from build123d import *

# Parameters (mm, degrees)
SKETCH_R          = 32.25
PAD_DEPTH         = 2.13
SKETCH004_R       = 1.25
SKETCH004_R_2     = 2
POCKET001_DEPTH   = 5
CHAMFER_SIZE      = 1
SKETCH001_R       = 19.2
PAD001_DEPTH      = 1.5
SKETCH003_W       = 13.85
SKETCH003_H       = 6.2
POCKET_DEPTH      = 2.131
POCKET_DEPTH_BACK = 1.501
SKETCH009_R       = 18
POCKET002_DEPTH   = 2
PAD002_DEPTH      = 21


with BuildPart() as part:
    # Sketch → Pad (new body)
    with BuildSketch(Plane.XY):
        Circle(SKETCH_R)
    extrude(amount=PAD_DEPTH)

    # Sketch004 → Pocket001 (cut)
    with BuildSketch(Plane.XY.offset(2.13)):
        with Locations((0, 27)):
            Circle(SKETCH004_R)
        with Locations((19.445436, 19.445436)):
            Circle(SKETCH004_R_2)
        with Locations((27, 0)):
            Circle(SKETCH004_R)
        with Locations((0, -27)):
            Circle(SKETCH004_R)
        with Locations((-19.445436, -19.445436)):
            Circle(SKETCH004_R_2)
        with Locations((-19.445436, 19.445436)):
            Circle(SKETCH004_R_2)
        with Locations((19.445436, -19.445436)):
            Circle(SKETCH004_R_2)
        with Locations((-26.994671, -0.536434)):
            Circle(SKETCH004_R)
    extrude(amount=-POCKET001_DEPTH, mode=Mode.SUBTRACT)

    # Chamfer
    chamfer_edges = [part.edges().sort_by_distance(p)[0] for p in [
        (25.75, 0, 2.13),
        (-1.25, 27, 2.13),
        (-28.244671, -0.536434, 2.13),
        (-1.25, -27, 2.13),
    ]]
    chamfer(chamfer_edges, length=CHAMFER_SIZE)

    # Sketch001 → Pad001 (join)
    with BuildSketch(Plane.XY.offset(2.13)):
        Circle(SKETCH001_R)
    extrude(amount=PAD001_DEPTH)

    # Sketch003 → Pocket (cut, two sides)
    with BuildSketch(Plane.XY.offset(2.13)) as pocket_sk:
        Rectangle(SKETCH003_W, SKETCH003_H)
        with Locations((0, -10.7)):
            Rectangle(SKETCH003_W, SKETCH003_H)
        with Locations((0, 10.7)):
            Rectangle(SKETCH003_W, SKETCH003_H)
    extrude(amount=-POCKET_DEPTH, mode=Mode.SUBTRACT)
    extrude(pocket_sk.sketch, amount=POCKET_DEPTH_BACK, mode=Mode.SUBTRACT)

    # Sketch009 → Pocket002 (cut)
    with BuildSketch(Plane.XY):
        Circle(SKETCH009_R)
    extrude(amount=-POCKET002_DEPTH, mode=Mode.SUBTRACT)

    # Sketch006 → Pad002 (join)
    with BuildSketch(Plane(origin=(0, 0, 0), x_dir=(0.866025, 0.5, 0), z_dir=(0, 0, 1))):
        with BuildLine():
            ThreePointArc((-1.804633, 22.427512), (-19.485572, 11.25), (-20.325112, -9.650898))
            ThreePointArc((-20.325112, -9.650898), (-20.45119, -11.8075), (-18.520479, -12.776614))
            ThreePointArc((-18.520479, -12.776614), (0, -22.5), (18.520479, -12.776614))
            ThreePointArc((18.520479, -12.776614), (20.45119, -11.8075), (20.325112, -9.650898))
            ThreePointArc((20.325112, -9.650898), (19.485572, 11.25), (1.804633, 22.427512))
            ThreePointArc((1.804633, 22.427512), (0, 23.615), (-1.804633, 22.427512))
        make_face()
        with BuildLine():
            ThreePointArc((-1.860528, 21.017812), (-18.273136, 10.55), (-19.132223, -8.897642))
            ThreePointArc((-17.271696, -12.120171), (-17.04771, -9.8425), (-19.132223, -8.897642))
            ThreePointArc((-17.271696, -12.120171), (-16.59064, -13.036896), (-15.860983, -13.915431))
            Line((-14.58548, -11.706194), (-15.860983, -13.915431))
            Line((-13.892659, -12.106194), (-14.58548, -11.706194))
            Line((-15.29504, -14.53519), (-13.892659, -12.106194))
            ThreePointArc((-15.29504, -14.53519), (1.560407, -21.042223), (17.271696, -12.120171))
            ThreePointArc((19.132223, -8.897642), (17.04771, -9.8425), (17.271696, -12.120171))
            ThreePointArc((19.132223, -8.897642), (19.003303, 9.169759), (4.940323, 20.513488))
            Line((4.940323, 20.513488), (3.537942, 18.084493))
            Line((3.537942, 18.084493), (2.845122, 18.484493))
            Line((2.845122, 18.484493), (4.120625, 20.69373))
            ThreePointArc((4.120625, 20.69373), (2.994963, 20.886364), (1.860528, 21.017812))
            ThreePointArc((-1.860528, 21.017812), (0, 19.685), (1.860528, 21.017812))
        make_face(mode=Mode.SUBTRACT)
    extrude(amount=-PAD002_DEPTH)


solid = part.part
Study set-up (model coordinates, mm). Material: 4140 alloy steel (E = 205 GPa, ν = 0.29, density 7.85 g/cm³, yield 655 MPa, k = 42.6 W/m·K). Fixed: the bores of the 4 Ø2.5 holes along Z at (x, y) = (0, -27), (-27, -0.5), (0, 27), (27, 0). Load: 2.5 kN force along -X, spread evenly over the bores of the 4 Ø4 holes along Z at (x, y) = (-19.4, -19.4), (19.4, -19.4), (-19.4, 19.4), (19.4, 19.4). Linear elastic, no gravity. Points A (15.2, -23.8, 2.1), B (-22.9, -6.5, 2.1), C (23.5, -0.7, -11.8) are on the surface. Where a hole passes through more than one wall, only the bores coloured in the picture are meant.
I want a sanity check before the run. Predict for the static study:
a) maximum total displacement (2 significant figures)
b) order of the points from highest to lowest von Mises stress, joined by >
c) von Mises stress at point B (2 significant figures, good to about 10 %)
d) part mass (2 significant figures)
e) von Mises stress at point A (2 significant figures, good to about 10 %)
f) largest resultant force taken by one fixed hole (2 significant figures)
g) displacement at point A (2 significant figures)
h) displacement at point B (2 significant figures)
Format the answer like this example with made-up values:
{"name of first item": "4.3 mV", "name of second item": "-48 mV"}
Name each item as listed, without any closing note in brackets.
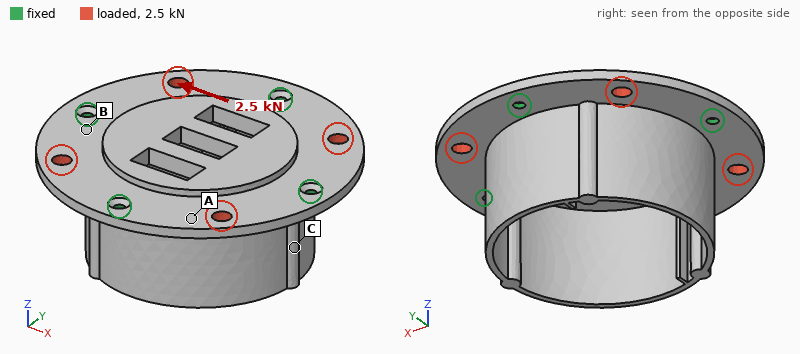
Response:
{"maximum total displacement": "3.0 µm", "order of the points from highest to lowest von Mises stress, joined by >": "A > B > C", "von Mises stress at point B": "11 MPa", "part mass": "95 g", "von Mises stress at point A": "21 MPa", "largest resultant force taken by one fixed hole": "760 N", "displacement at point A": "1.9 µm", "displacement at point B": "1.0 µm"}
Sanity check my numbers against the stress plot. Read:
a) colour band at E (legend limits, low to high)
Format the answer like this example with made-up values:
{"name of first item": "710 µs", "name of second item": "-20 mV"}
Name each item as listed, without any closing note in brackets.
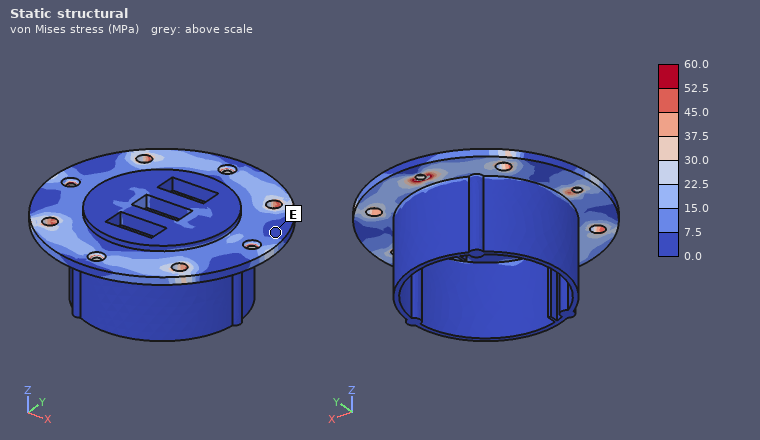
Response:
{"colour band at E": "0.0 to 7.5 MPa"}
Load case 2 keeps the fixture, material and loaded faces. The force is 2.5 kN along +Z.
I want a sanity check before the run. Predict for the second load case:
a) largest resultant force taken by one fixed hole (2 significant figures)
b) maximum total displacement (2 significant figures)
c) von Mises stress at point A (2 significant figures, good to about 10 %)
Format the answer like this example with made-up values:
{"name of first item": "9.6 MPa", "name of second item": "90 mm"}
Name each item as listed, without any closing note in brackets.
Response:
{"largest resultant force taken by one fixed hole": "650 N", "maximum total displacement": "61 µm", "von Mises stress at point A": "82 MPa"}
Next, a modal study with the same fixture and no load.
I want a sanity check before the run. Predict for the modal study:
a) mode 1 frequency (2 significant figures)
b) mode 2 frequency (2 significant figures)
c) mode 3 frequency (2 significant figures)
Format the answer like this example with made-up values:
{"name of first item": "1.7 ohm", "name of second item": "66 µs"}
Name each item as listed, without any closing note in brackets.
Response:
{"mode 1 frequency": "4000 Hz", "mode 2 frequency": "6100 Hz", "mode 3 frequency": "6300 Hz"}
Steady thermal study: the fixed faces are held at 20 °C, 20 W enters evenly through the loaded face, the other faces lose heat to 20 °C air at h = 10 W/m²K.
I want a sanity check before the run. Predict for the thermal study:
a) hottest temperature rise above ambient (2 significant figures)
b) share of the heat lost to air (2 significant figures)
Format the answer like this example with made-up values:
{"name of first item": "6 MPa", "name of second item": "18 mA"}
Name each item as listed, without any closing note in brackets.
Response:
{"hottest temperature rise above ambient": "49 K", "share of the heat lost to air": "15 %"}
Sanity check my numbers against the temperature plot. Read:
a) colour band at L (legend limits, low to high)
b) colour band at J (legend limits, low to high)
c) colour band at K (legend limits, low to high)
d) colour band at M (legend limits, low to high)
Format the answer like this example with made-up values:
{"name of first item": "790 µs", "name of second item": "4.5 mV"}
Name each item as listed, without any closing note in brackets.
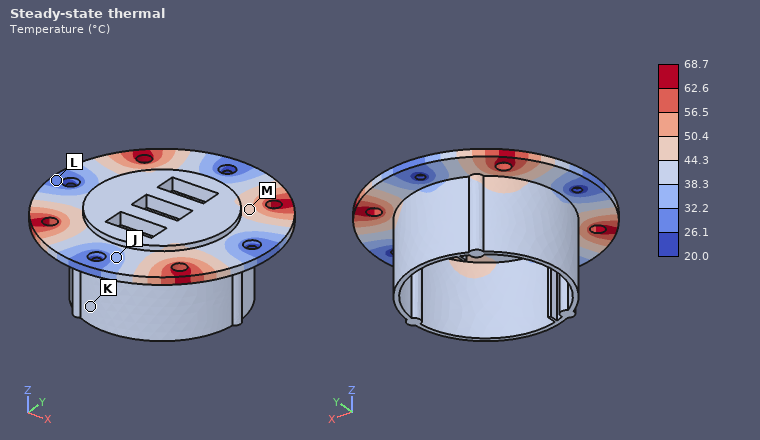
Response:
{"colour band at L": "26.1 to 32.2 °C", "colour band at J": "32.2 to 38.3 °C", "colour band at K": "38.3 to 44.3 °C", "colour band at M": "44.3 to 50.4 °C"}
